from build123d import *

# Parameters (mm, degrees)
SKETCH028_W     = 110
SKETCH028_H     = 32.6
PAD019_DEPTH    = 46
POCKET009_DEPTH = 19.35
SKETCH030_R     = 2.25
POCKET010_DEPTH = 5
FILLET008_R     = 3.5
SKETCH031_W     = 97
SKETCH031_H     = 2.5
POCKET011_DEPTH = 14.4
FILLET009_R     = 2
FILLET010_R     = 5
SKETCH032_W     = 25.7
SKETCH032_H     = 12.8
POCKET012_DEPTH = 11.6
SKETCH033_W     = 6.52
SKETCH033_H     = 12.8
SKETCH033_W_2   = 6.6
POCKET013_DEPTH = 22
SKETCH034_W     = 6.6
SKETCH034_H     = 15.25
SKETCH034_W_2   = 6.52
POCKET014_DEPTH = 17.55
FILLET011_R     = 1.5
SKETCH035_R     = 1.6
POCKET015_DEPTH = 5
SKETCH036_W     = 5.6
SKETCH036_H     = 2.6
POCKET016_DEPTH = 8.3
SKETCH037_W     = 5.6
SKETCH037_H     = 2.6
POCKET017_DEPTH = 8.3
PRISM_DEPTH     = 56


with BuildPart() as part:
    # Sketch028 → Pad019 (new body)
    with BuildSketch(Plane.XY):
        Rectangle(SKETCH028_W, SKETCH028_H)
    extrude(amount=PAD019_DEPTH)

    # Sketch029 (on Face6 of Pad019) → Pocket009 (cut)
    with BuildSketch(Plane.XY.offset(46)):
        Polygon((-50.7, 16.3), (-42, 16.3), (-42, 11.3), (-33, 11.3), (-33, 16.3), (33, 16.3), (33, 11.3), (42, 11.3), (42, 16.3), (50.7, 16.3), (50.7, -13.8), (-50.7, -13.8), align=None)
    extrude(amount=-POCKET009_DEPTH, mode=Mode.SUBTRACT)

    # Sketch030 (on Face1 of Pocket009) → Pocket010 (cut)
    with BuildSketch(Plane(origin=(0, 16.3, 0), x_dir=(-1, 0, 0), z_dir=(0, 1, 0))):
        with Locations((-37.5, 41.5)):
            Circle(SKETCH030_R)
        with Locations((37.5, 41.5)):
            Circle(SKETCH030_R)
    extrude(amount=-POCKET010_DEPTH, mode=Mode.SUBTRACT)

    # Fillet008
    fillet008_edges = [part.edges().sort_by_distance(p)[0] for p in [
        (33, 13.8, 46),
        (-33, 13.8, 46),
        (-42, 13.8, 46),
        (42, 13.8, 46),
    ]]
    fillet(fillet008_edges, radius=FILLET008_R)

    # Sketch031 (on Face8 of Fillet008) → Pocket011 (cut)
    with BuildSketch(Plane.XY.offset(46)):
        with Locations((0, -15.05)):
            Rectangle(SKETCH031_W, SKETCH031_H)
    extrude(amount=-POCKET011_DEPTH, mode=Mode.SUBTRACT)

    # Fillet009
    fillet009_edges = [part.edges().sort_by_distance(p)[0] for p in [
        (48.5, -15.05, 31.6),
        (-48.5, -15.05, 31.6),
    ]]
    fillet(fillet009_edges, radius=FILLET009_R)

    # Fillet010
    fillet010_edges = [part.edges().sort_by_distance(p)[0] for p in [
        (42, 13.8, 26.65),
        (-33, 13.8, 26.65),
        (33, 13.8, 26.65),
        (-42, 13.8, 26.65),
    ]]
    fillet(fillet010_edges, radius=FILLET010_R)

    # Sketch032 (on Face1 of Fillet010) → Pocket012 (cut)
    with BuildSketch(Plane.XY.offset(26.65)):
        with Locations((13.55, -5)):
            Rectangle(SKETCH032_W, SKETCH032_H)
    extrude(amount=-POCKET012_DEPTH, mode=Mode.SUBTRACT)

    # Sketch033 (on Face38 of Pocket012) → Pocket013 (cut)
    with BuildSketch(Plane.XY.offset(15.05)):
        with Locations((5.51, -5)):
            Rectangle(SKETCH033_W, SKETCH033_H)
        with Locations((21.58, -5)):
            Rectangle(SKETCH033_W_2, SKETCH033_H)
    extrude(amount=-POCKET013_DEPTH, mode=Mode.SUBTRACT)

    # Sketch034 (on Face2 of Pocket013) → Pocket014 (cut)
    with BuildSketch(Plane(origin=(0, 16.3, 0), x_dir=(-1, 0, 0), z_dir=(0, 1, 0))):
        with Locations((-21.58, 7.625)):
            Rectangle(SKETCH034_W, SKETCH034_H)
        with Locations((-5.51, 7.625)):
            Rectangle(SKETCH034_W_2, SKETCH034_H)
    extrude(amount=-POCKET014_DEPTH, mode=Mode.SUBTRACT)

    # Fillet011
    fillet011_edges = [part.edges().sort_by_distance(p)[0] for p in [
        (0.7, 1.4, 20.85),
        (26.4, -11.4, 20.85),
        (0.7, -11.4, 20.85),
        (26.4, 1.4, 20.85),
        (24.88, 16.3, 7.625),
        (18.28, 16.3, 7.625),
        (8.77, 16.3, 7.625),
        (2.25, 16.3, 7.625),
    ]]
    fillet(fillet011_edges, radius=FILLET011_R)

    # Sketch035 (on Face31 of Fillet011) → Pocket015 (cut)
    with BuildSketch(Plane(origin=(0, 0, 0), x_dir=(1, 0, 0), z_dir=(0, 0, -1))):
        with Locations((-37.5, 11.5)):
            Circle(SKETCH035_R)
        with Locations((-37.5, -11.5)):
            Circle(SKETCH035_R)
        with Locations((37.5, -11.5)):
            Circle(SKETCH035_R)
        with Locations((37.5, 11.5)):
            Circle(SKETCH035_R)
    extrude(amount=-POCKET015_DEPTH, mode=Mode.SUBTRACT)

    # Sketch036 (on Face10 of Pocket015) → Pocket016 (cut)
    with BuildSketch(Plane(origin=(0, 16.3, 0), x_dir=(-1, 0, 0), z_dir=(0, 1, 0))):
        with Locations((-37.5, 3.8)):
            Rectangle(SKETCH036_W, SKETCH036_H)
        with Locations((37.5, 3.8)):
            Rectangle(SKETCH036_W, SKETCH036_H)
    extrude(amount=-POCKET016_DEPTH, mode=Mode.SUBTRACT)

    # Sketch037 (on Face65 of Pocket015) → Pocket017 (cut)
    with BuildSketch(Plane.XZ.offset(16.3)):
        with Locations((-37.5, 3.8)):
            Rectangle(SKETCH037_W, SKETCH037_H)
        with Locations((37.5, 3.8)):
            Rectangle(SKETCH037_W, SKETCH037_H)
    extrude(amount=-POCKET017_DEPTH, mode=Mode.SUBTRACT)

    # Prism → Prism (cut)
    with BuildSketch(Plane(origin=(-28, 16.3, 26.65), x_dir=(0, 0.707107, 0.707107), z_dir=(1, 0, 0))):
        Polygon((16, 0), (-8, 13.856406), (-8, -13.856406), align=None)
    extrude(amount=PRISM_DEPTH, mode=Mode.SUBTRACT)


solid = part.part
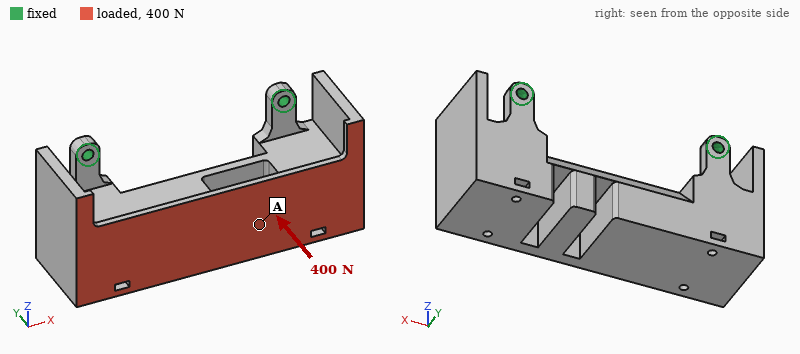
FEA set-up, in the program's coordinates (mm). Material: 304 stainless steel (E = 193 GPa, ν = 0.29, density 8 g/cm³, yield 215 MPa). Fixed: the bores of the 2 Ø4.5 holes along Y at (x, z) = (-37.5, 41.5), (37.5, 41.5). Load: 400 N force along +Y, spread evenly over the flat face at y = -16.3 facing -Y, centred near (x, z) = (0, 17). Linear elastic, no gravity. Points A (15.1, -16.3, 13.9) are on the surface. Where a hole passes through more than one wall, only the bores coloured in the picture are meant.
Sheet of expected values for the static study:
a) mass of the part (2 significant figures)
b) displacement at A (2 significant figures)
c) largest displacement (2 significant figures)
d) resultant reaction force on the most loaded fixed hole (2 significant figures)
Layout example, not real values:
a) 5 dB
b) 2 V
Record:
a) 720 g
b) 0.090 mm
c) 0.11 mm
d) 200 N
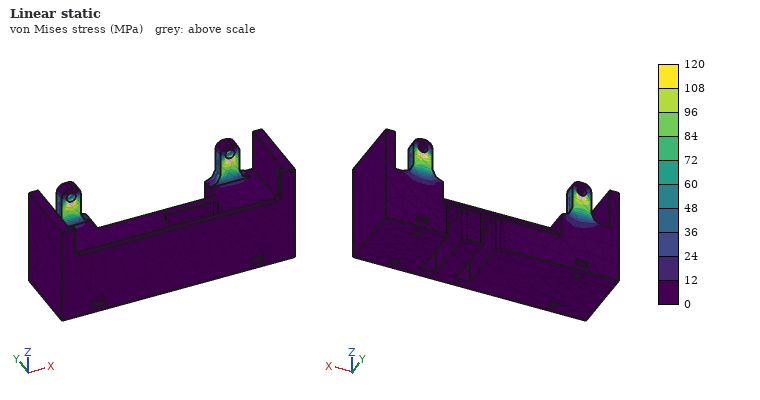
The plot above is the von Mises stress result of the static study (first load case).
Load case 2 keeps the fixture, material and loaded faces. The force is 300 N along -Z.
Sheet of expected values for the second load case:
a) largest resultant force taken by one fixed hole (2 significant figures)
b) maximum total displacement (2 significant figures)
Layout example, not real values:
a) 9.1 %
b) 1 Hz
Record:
a) 150 N
b) 0.16 mm
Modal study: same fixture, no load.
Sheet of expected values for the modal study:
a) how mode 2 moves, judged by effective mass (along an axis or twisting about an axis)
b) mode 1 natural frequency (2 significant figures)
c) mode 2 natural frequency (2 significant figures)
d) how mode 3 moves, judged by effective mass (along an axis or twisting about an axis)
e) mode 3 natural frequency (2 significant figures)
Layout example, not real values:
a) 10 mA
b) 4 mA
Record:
a) along X
b) 350 Hz
c) 1600 Hz
d) along X
e) 2300 Hz
